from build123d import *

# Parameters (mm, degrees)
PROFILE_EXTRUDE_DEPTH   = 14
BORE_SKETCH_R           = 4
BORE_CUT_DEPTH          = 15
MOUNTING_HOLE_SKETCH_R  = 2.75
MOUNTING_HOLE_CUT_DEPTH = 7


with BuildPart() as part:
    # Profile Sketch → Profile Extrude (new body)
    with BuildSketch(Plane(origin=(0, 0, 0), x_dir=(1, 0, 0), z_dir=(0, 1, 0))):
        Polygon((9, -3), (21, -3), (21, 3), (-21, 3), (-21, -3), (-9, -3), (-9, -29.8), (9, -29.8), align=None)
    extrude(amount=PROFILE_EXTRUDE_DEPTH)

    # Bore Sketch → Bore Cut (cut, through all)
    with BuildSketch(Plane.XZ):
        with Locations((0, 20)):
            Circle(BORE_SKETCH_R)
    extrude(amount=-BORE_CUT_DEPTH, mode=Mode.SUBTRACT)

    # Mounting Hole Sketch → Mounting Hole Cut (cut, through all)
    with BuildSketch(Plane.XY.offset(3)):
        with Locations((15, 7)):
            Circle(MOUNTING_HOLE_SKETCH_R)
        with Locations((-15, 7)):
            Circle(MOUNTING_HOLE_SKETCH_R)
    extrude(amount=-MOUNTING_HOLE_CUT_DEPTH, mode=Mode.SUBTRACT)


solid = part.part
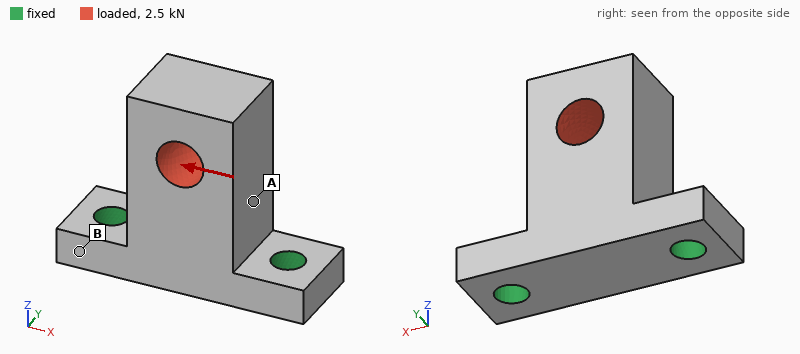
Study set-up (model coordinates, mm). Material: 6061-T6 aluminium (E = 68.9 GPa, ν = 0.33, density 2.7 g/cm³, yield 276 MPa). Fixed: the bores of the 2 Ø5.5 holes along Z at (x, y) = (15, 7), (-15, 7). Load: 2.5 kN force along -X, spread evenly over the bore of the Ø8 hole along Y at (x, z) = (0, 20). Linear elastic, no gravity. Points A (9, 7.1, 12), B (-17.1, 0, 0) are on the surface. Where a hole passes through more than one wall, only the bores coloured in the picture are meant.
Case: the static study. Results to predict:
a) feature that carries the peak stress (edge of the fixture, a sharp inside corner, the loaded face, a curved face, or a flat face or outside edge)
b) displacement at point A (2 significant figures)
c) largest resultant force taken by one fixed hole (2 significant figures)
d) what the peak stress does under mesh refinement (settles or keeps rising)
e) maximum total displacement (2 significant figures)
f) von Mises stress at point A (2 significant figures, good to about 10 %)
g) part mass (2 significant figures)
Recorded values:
edge of the fixture
25 µm
2.5 kN
keeps rising
63 µm
34 MPa
25 g
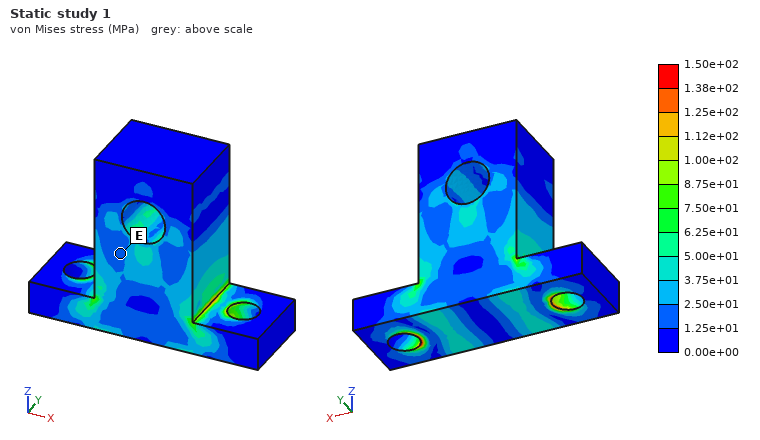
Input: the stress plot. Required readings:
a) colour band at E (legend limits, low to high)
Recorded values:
1.25e+01 to 2.50e+01 MPa
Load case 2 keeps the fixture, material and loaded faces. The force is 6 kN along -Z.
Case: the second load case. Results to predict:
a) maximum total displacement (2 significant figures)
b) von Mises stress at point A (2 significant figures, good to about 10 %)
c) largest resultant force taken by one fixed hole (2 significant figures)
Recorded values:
28 µm
30 MPa
3.2 kN
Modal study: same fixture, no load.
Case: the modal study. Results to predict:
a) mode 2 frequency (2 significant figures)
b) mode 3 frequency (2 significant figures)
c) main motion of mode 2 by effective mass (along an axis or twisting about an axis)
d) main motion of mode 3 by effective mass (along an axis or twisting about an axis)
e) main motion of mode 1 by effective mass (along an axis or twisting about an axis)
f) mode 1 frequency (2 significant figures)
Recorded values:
11 kHz
19 kHz
along X
along Z
along Y
5200 Hz
